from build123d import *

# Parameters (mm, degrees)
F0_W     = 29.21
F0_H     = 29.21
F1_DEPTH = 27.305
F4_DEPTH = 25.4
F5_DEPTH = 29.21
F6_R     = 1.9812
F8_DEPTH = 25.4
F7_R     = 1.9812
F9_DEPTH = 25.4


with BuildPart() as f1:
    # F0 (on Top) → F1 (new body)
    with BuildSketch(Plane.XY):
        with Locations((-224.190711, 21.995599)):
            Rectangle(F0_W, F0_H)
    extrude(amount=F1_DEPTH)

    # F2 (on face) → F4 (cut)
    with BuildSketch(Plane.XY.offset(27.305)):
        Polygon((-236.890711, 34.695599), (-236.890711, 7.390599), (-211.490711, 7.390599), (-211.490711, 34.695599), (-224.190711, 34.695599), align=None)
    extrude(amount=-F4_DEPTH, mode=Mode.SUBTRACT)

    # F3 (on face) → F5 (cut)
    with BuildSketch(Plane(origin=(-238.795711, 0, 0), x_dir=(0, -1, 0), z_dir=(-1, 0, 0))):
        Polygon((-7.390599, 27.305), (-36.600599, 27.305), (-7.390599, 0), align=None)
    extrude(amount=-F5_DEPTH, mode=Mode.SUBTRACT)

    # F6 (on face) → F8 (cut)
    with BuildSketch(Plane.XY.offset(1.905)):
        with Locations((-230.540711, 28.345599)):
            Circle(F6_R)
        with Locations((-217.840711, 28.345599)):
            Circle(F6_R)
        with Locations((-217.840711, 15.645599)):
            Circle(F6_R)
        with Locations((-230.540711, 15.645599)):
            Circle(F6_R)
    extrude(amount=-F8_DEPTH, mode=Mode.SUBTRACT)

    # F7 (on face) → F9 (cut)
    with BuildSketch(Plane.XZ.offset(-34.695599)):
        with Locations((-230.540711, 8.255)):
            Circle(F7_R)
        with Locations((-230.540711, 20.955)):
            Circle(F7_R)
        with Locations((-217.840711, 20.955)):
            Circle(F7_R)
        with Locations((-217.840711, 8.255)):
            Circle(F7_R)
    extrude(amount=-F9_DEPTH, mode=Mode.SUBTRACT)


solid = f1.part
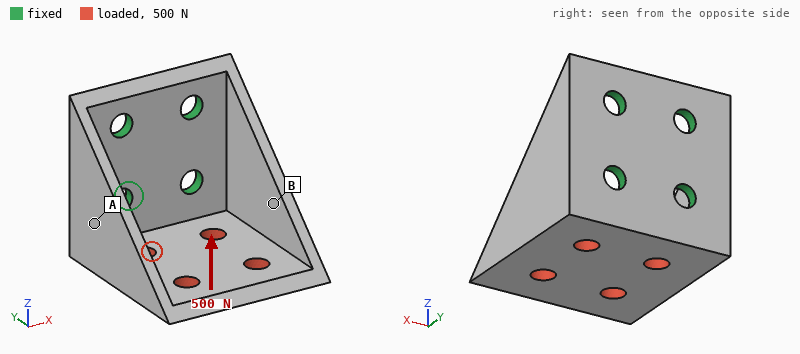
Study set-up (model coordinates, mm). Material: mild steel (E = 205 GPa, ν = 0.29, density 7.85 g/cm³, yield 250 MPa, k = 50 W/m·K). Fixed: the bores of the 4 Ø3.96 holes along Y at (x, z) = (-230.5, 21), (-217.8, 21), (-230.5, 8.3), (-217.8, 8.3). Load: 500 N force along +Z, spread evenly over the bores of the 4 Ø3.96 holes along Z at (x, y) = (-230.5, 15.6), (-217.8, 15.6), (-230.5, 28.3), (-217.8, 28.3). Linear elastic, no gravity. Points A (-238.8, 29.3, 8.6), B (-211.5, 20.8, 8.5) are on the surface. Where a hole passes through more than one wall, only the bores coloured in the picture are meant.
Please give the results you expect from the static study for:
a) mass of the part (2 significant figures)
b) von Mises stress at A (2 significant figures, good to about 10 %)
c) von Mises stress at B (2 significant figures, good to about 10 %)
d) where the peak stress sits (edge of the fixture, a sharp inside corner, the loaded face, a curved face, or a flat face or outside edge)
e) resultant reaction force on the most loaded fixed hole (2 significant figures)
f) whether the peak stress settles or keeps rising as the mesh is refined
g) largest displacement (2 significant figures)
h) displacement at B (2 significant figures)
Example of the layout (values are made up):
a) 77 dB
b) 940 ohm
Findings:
a) 30 g
b) 19 MPa
c) 44 MPa
d) edge of the fixture
e) 270 N
f) keeps rising
g) 60 µm
h) 20 µm
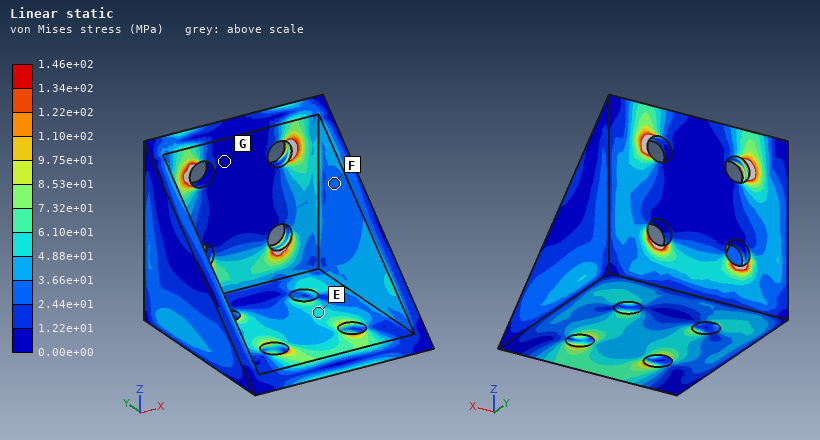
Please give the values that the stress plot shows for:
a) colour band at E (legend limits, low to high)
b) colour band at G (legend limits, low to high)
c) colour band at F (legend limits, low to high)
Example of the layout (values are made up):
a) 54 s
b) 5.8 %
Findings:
a) 4.88e+01 to 6.10e+01 MPa
b) 0.00e+00 to 1.22e+01 MPa
c) 2.44e+01 to 3.66e+01 MPa
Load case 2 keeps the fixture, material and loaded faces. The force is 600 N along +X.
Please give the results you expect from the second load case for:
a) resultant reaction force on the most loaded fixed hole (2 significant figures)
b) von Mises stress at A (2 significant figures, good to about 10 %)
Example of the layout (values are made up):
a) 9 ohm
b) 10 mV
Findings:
a) 620 N
b) 21 MPa
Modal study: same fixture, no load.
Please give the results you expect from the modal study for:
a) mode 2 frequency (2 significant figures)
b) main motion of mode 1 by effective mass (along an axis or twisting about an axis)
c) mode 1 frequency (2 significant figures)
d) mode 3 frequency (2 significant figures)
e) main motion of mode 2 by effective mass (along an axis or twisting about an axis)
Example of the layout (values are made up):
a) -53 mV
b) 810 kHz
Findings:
a) 5300 Hz
b) along X
c) 4800 Hz
d) 11 kHz
e) along Z
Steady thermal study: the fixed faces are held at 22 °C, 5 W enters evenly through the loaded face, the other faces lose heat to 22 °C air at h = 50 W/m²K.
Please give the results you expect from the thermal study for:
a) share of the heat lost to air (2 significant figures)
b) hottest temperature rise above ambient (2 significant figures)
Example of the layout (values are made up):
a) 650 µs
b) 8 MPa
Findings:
a) 32 %
b) 19 K
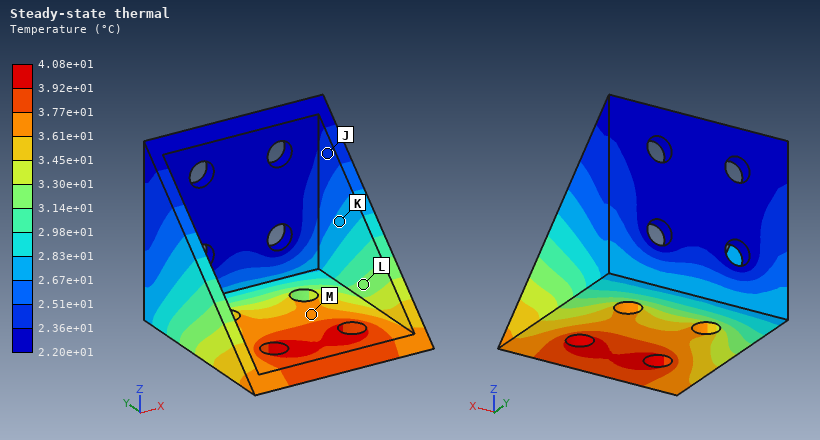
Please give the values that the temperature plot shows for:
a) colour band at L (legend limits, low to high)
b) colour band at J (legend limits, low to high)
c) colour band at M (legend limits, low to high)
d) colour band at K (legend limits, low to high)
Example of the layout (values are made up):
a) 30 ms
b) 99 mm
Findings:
a) 3.14e+01 to 3.30e+01 °C
b) 2.36e+01 to 2.51e+01 °C
c) 3.61e+01 to 3.77e+01 °C
d) 2.67e+01 to 2.83e+01 °C
